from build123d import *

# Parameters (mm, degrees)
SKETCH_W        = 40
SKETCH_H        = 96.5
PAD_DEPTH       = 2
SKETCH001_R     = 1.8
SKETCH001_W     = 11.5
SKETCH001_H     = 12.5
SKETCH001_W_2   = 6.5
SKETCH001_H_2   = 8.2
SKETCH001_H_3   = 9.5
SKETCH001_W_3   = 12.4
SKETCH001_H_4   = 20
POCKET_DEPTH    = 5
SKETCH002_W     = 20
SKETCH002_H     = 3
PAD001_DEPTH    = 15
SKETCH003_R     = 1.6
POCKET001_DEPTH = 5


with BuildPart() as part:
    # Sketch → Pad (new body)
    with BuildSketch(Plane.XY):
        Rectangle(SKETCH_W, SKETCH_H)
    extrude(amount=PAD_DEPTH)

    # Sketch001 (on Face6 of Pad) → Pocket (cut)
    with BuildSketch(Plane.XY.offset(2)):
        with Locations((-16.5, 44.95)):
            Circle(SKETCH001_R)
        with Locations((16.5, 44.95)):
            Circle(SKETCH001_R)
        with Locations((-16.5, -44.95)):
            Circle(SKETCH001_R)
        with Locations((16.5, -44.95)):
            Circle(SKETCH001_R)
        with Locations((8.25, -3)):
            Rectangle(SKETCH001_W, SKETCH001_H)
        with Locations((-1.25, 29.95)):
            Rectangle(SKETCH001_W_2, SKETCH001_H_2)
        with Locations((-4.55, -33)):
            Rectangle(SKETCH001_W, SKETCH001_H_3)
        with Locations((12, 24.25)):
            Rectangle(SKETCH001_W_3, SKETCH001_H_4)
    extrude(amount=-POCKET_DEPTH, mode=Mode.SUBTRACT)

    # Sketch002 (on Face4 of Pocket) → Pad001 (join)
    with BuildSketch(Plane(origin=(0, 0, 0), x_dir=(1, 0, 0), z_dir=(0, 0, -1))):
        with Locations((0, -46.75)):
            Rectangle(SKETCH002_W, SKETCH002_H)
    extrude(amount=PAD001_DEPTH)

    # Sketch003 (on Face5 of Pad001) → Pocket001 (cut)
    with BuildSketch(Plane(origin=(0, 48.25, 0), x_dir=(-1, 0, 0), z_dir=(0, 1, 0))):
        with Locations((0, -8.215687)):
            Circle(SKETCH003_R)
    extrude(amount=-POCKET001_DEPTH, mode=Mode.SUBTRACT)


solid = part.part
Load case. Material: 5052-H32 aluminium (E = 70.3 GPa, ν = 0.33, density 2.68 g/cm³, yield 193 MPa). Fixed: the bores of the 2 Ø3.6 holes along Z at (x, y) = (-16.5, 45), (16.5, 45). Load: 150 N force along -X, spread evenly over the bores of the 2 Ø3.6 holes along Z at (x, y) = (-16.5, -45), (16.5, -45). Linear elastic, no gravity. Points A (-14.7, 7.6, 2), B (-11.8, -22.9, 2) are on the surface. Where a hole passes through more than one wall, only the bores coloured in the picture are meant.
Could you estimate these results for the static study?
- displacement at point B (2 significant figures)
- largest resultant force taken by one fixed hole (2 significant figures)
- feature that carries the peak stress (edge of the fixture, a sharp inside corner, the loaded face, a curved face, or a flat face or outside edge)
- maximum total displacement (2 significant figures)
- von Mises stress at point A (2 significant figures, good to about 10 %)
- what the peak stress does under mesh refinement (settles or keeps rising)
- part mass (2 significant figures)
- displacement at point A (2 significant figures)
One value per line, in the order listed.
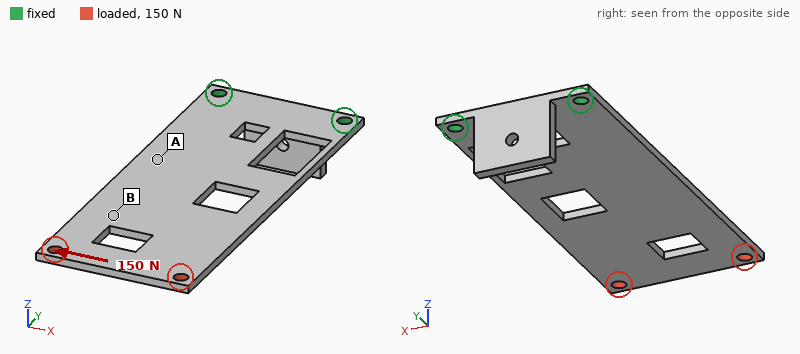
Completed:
0.070 mm
420 N
a sharp inside corner
0.11 mm
12 MPa
keeps rising
20 g
0.031 mm
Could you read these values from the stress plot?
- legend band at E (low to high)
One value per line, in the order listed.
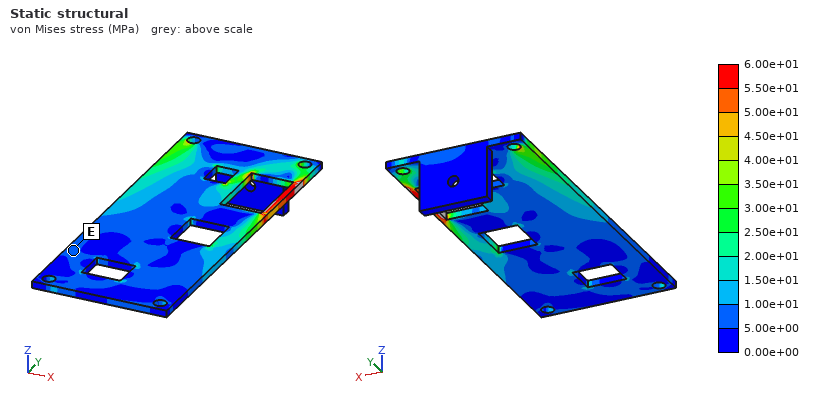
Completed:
5.00e+00 to 1.00e+01 MPa
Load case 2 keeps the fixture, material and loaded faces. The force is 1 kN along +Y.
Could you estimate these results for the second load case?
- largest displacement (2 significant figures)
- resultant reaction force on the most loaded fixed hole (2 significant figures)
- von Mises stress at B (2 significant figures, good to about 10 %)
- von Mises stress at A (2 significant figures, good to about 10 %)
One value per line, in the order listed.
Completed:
71 µm
520 N
20 MPa
13 MPa
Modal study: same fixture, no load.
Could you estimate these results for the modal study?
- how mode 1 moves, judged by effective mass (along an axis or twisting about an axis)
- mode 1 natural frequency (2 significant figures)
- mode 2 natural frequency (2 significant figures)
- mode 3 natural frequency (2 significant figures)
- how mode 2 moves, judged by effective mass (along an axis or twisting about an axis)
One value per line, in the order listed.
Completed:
along Z
160 Hz
830 Hz
1100 Hz
twisting about Y
